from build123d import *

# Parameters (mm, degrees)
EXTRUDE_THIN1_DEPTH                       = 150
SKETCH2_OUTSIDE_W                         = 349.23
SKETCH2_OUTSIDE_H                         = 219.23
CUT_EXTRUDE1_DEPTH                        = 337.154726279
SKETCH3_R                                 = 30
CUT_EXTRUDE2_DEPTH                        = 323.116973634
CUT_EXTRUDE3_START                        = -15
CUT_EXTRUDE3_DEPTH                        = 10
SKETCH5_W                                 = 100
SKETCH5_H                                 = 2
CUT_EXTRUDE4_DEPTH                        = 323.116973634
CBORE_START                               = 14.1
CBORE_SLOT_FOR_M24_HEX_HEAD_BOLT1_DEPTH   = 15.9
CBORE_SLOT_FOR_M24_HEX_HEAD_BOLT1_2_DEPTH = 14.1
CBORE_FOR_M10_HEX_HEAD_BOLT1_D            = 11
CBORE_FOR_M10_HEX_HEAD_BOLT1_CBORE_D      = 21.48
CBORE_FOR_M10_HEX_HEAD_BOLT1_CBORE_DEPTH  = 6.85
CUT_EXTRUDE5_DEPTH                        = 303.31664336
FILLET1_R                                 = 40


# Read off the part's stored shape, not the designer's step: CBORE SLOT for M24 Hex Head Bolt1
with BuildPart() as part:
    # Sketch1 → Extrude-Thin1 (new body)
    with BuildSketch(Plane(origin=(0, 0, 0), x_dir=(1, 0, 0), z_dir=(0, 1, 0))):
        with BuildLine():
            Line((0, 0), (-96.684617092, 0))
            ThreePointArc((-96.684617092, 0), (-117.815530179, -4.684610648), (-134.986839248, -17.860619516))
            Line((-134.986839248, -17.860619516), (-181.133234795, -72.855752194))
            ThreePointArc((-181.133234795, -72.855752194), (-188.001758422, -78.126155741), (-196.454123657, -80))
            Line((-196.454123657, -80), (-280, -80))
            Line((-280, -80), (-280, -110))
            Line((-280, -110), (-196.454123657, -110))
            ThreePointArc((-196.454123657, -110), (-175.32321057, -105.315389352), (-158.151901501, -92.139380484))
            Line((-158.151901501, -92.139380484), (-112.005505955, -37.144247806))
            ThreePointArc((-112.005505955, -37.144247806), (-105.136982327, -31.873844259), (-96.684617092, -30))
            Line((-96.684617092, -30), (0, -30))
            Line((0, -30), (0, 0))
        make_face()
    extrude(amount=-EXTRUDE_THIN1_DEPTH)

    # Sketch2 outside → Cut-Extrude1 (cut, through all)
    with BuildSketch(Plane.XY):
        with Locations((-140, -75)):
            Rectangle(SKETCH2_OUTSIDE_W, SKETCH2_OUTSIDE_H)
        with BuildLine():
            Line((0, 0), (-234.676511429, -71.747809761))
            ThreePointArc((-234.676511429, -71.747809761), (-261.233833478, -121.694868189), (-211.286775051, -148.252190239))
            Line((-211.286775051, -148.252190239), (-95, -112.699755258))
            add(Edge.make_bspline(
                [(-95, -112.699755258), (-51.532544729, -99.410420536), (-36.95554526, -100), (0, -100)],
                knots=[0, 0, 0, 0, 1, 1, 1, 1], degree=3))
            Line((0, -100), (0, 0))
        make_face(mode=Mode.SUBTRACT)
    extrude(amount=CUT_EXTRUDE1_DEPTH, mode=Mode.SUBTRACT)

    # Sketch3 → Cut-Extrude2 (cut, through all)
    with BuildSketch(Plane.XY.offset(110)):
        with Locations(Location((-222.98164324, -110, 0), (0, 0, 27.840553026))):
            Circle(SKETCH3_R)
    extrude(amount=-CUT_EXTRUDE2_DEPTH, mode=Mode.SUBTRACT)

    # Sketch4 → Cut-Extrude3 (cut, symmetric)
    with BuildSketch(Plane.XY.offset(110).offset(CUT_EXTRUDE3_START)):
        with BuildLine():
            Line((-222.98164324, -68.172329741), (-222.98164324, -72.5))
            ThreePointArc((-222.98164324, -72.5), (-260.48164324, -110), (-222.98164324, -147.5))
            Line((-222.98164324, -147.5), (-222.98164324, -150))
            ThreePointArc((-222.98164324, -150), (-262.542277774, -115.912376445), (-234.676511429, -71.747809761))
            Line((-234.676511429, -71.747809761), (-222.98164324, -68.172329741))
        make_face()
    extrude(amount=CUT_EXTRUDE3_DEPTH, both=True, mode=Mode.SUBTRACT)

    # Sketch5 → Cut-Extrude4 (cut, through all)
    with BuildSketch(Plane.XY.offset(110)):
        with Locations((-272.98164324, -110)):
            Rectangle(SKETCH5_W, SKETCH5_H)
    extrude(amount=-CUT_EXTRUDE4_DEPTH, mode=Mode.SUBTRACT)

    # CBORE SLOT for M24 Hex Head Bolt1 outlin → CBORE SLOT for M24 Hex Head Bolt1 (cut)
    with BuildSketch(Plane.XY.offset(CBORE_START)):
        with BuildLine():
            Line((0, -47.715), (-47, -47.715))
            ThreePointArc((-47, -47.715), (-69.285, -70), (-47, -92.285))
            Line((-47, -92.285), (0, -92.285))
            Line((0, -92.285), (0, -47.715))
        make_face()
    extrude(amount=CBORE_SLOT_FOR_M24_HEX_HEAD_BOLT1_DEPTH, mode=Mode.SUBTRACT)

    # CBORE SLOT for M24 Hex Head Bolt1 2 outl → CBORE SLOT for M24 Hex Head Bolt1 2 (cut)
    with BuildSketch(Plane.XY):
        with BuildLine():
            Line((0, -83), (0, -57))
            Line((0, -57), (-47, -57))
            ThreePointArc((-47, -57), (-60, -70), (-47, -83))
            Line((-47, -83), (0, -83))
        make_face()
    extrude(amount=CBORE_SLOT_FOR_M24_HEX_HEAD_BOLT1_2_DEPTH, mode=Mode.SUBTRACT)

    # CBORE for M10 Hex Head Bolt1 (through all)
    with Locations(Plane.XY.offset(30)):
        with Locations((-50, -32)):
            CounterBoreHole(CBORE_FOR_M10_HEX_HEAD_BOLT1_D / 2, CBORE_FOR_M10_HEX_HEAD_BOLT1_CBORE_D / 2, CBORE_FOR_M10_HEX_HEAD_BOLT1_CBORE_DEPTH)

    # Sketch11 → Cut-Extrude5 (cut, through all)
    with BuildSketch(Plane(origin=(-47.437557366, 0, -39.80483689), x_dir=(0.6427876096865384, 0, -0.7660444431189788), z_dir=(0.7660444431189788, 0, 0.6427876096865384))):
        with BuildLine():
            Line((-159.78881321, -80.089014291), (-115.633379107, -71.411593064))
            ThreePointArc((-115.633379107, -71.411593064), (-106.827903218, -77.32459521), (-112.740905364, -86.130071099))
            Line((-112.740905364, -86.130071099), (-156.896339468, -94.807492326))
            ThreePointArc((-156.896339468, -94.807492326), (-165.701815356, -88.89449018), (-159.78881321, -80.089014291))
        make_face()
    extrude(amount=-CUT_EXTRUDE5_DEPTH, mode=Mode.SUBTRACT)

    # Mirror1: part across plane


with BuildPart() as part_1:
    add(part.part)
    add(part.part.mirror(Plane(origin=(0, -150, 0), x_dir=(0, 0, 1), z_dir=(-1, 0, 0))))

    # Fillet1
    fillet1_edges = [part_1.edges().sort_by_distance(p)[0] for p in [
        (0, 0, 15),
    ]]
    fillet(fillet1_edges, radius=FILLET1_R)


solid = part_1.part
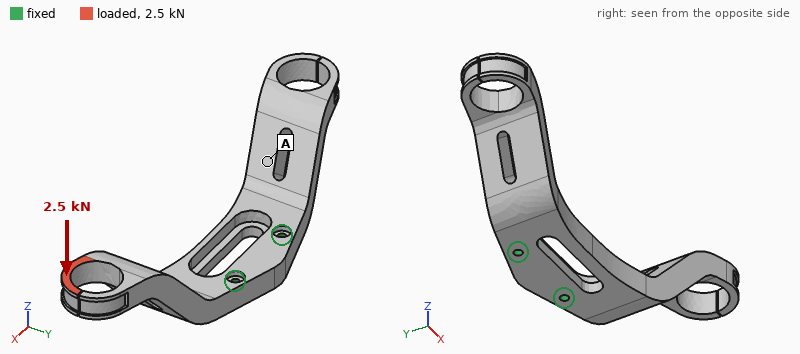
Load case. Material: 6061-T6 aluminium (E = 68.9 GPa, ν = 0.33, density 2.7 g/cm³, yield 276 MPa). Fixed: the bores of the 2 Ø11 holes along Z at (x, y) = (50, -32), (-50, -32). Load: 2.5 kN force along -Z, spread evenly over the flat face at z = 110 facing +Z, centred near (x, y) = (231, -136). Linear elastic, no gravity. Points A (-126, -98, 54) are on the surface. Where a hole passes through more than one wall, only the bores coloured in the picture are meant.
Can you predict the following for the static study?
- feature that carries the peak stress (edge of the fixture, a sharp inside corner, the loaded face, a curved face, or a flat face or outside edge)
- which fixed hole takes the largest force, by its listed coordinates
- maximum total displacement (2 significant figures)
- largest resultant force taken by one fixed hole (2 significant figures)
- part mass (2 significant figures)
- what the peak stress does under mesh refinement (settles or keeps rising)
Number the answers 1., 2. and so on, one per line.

1. edge of the fixture
2. (50, -32)
3. 1.6 mm
4. 4.4 kN
5. 2.9 kg
6. keeps rising
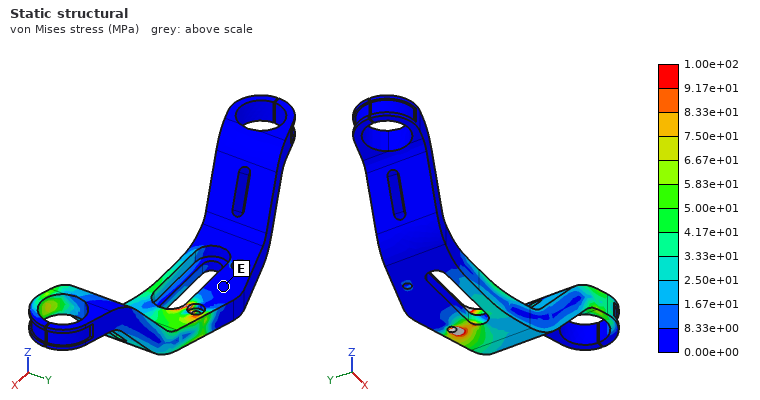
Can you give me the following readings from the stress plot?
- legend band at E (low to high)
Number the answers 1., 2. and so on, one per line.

1. 0.00e+00 to 8.33e+00 MPa
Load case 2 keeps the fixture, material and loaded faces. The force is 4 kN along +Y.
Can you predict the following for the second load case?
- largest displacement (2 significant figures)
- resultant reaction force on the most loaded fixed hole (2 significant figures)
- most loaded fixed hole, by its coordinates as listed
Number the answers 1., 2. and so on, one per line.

1. 2.2 mm
2. 9.8 kN
3. (50, -32)
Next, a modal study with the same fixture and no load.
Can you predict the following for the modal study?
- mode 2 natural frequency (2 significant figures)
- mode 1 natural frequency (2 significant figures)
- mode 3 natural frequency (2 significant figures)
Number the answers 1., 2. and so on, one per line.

1. 400 Hz
2. 390 Hz
3. 520 Hz
